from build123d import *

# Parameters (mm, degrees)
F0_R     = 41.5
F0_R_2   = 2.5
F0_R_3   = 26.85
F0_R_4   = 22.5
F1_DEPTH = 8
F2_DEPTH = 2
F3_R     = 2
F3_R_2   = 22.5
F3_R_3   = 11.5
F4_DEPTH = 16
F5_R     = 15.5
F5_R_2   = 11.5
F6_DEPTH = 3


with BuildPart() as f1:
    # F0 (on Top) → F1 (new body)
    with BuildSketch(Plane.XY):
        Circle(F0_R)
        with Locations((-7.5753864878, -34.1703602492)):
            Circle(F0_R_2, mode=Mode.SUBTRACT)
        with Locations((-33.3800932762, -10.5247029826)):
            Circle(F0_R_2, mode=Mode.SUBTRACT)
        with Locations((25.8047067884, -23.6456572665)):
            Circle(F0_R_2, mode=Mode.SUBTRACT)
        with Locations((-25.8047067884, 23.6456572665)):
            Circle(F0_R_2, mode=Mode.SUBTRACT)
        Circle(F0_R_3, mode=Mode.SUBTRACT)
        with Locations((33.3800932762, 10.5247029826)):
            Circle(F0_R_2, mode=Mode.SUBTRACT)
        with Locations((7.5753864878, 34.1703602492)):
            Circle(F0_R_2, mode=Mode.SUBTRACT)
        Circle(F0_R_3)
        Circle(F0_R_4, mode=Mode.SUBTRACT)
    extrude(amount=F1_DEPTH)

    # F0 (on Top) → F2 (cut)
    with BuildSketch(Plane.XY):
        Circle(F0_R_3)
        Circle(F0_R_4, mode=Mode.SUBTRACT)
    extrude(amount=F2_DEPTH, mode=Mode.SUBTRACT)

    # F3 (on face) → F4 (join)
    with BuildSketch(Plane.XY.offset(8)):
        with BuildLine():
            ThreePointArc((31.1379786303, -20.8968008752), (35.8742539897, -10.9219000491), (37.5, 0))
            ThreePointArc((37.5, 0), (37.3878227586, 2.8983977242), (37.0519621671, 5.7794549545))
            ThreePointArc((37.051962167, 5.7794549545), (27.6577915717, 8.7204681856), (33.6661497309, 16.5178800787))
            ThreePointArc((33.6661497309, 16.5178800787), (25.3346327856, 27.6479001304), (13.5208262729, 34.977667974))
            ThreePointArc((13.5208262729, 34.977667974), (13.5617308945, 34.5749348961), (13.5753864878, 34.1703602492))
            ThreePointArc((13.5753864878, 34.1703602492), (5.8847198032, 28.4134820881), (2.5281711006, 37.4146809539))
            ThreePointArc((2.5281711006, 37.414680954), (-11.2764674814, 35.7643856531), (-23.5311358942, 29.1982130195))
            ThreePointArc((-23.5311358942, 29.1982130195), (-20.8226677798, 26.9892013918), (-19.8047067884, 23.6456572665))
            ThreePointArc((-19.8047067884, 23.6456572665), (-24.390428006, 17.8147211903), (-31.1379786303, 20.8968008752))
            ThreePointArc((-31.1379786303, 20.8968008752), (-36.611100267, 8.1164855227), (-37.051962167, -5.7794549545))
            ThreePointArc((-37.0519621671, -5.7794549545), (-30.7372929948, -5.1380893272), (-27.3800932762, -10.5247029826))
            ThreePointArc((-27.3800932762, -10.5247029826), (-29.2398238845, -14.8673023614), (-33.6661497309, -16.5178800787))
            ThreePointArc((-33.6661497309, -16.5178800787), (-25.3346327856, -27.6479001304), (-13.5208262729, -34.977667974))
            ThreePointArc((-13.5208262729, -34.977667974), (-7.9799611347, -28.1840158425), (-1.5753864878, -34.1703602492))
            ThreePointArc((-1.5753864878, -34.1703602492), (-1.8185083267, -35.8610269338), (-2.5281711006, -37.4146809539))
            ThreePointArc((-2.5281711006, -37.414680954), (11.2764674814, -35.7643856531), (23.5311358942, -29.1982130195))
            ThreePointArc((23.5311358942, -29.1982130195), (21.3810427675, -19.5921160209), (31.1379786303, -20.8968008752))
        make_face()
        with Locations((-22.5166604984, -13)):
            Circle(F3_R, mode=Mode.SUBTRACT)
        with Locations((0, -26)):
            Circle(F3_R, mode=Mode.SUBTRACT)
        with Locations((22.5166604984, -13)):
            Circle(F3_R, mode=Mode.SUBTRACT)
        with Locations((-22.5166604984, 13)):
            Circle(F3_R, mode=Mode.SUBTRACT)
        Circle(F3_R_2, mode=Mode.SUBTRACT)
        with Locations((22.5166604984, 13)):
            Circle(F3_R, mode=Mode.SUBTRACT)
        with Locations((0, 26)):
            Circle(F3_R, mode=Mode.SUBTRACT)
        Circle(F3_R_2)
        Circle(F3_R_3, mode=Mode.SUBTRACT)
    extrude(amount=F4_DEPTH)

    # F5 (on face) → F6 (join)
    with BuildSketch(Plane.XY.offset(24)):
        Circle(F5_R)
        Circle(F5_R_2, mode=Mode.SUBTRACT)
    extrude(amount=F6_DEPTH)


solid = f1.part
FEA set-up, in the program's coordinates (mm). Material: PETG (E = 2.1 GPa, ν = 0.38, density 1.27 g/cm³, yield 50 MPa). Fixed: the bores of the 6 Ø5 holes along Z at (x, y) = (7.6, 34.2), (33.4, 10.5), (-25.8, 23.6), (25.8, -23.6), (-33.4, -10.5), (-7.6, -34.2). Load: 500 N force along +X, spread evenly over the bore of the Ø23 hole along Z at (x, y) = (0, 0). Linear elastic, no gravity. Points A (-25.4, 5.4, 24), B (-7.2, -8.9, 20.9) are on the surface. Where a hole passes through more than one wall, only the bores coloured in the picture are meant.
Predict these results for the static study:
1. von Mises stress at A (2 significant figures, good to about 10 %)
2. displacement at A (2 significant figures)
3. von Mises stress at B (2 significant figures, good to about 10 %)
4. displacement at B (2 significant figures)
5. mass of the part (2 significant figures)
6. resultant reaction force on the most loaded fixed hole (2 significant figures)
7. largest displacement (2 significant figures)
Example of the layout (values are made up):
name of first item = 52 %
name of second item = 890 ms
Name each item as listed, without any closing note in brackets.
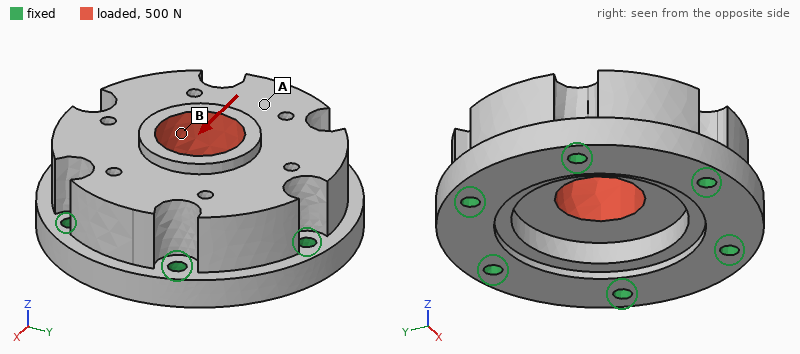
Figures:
von Mises stress at A = 0.30 MPa
displacement at A = 12 µm
von Mises stress at B = 0.81 MPa
displacement at B = 13 µm
mass of the part = 110 g
resultant reaction force on the most loaded fixed hole = 110 N
largest displacement = 18 µm
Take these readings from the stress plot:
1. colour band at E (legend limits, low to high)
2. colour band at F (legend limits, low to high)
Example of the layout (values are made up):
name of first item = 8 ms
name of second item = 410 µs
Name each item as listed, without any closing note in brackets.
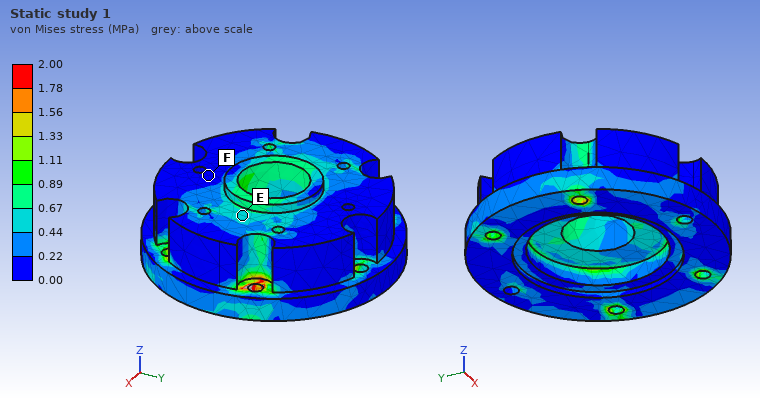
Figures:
colour band at E = 0.44 to 0.67 MPa
colour band at F = 0.00 to 0.22 MPa
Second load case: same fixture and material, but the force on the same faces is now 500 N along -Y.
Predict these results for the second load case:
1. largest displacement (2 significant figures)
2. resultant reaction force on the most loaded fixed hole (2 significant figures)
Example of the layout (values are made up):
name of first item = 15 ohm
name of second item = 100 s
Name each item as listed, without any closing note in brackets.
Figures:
largest displacement = 18 µm
resultant reaction force on the most loaded fixed hole = 120 N
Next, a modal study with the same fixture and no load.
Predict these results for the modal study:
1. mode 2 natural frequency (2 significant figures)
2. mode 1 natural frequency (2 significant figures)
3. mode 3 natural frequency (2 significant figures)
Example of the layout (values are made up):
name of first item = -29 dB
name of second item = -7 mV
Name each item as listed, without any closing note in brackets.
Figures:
mode 2 natural frequency = 4500 Hz
mode 1 natural frequency = 4400 Hz
mode 3 natural frequency = 4500 Hz
